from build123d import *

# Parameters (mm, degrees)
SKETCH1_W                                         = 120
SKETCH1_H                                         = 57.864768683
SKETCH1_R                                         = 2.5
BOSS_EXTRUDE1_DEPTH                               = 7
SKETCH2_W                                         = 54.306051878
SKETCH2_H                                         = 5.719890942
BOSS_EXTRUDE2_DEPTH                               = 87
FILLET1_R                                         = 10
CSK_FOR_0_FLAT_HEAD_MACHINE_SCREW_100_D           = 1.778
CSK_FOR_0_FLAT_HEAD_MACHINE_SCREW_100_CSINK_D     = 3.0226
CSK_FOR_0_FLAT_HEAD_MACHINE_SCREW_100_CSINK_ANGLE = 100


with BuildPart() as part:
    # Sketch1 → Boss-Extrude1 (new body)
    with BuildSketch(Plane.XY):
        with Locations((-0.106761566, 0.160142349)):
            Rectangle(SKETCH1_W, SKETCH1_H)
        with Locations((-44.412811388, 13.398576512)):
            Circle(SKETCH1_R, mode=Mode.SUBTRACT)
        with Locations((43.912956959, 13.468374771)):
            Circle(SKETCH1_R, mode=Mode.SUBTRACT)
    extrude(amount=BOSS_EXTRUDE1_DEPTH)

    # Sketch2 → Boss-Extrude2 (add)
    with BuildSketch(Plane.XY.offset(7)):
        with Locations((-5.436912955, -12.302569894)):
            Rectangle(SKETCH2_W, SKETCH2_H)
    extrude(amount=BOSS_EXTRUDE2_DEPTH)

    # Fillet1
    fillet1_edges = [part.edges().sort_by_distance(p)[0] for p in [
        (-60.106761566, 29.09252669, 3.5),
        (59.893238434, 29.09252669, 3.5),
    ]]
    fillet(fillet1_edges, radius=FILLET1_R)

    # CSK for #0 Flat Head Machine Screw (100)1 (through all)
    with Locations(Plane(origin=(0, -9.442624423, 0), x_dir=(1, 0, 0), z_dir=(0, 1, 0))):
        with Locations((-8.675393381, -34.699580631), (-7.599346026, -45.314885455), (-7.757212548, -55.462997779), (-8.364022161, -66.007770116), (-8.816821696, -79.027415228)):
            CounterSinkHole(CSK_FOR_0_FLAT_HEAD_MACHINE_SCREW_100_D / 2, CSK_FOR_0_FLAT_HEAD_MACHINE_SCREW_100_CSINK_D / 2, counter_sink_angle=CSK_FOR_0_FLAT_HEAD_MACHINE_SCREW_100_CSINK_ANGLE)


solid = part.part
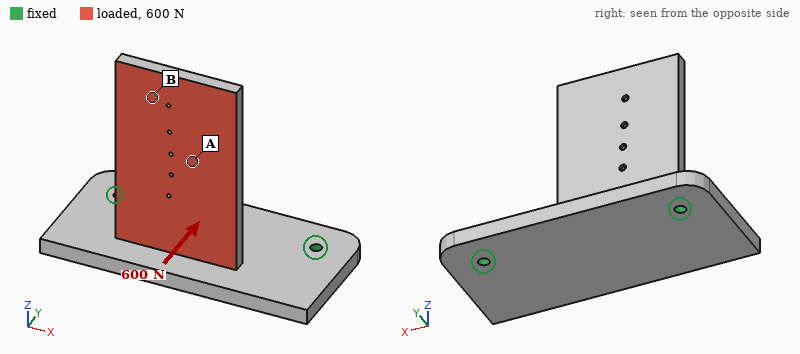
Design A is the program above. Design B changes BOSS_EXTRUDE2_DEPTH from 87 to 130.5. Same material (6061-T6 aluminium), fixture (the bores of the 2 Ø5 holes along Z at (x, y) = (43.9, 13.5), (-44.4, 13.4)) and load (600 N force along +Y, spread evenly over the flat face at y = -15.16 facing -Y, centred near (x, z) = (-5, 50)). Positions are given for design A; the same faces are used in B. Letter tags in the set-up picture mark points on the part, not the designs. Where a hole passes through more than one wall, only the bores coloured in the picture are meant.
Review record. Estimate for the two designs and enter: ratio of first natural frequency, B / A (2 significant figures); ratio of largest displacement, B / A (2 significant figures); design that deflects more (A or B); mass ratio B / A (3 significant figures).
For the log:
0.48
2.9
B
1.18
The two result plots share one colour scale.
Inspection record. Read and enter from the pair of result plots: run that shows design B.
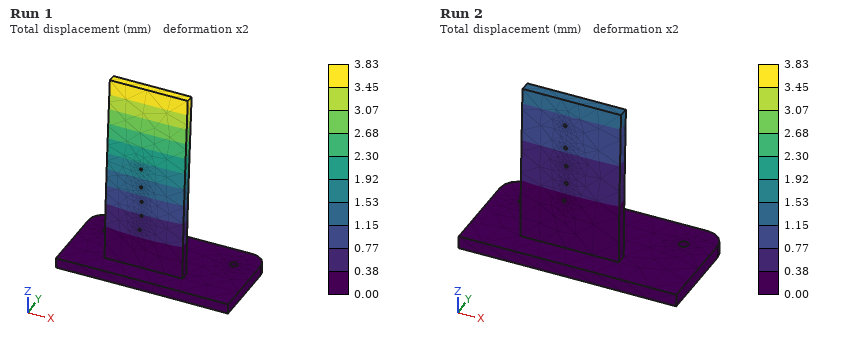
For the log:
Run 1
